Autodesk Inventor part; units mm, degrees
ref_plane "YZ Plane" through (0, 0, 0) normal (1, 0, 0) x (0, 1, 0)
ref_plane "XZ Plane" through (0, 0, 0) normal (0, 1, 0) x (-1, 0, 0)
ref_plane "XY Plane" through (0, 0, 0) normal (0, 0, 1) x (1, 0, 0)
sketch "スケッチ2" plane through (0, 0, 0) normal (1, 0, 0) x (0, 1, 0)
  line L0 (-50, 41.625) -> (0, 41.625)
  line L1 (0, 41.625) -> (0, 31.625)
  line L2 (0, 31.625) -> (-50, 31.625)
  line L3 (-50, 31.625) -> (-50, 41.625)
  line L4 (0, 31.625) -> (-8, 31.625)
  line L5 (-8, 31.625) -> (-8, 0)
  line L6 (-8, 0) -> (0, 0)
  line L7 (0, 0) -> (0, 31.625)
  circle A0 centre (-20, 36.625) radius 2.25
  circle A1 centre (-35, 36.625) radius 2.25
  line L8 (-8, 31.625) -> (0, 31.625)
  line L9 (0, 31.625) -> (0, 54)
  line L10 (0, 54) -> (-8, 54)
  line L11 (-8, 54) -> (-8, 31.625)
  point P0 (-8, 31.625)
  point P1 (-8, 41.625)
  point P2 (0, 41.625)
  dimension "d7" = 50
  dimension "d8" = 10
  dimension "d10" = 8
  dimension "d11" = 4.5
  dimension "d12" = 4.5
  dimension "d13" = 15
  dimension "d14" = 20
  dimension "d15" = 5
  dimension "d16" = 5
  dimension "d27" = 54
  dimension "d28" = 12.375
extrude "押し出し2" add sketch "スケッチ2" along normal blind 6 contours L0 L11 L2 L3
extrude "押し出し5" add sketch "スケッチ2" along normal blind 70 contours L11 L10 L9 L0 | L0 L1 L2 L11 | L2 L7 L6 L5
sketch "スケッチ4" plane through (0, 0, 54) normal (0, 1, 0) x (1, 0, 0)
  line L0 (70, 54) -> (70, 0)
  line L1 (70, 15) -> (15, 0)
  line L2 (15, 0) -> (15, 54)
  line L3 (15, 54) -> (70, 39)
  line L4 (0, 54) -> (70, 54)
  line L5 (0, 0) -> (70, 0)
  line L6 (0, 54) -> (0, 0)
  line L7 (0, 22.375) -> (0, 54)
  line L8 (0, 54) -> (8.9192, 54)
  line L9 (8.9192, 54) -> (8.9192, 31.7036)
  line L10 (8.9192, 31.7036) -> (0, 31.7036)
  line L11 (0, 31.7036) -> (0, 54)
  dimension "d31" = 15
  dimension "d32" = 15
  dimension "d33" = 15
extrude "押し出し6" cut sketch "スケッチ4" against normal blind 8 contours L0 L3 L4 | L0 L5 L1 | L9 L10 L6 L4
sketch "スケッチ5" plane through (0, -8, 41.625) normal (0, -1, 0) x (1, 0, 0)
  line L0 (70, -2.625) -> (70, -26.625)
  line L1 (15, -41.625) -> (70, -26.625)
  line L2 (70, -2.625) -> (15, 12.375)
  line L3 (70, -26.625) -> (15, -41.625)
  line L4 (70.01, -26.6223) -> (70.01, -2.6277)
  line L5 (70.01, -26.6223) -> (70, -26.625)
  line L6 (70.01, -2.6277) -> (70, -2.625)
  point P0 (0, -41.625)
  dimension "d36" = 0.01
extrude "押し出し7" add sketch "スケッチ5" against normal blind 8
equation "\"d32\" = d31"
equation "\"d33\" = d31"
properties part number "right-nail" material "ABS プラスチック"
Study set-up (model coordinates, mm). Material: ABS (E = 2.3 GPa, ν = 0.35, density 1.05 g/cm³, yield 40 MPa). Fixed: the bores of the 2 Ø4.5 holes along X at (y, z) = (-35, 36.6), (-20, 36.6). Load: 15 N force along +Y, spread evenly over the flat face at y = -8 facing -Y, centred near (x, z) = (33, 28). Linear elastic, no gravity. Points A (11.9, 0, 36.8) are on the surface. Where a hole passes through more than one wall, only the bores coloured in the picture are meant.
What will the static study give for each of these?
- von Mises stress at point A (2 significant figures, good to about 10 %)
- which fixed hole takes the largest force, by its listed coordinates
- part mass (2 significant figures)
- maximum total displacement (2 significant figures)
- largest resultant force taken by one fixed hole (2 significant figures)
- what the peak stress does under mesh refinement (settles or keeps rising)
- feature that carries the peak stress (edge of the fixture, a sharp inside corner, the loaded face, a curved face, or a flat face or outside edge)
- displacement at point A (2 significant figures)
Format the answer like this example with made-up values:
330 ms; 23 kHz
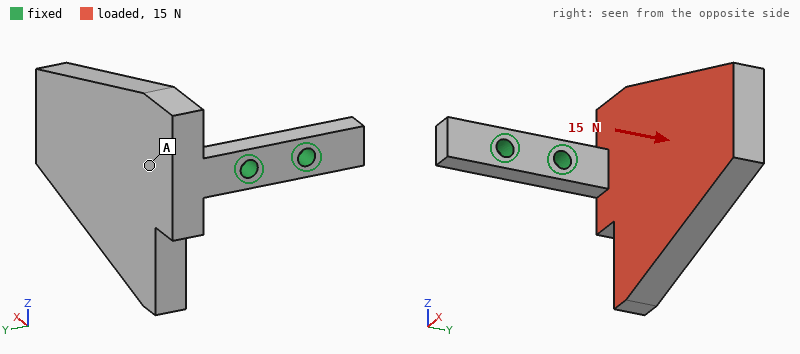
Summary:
1.1 MPa; (-20, 36.6); 26 g; 1.1 mm; 15 N; keeps rising; edge of the fixture; 0.22 mm
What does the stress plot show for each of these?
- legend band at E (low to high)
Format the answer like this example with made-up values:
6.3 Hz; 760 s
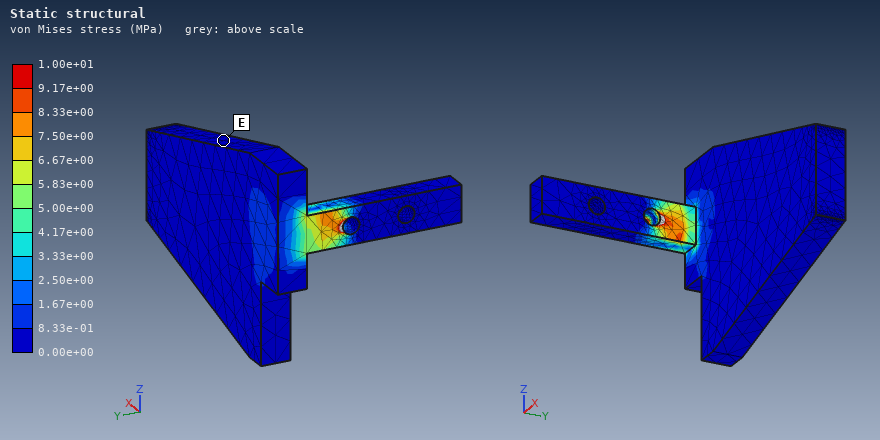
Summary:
0.00e+00 to 8.33e-01 MPa
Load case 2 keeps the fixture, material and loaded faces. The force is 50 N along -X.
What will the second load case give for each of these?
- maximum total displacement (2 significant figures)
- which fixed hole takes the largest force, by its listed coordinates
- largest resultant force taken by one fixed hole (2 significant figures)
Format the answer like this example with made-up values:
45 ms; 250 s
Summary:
1.0 mm; (-20, 36.6); 53 N
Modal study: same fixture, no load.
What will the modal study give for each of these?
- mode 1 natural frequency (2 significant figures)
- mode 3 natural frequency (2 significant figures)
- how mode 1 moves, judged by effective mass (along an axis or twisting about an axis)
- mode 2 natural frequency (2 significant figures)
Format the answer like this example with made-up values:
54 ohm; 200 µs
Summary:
150 Hz; 550 Hz; along Y; 160 Hz
